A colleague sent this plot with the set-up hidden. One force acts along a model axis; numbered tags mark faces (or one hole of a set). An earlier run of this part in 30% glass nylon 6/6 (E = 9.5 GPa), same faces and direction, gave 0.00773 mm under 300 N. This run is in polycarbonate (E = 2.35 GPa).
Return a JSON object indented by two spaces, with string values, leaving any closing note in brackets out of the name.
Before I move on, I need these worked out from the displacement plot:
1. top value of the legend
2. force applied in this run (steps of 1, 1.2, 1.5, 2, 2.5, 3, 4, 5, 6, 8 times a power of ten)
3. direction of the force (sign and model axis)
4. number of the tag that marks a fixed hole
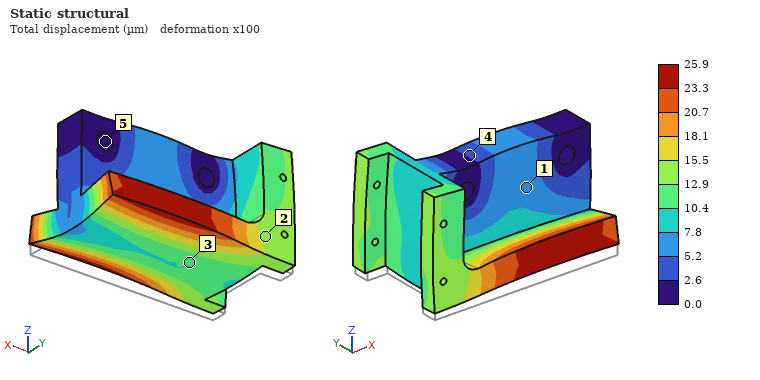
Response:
{
  "top value of the legend": "25.9 µm",
  "force applied in this run": "250 N",
  "direction of the force": "+Z",
  "number of the tag that marks a fixed hole": "5"
}
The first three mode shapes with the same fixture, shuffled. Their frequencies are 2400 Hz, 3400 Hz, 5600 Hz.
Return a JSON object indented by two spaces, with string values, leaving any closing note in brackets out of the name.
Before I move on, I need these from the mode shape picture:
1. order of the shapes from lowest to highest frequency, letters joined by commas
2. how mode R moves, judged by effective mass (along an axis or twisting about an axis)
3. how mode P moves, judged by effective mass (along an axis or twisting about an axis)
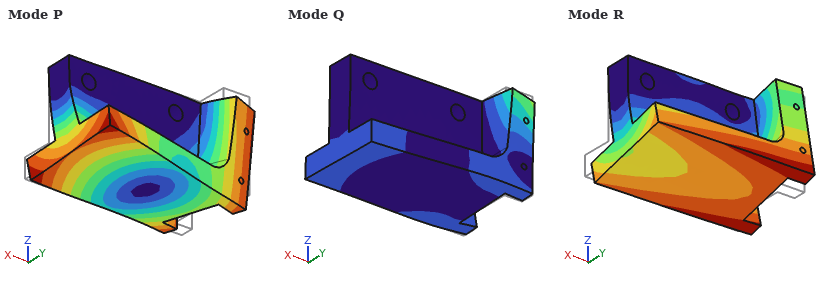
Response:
{
  "order of the shapes from lowest to highest frequency, letters joined by commas": "R, P, Q",
  "how mode R moves, judged by effective mass": "along Y",
  "how mode P moves, judged by effective mass": "twisting about Z"
}
